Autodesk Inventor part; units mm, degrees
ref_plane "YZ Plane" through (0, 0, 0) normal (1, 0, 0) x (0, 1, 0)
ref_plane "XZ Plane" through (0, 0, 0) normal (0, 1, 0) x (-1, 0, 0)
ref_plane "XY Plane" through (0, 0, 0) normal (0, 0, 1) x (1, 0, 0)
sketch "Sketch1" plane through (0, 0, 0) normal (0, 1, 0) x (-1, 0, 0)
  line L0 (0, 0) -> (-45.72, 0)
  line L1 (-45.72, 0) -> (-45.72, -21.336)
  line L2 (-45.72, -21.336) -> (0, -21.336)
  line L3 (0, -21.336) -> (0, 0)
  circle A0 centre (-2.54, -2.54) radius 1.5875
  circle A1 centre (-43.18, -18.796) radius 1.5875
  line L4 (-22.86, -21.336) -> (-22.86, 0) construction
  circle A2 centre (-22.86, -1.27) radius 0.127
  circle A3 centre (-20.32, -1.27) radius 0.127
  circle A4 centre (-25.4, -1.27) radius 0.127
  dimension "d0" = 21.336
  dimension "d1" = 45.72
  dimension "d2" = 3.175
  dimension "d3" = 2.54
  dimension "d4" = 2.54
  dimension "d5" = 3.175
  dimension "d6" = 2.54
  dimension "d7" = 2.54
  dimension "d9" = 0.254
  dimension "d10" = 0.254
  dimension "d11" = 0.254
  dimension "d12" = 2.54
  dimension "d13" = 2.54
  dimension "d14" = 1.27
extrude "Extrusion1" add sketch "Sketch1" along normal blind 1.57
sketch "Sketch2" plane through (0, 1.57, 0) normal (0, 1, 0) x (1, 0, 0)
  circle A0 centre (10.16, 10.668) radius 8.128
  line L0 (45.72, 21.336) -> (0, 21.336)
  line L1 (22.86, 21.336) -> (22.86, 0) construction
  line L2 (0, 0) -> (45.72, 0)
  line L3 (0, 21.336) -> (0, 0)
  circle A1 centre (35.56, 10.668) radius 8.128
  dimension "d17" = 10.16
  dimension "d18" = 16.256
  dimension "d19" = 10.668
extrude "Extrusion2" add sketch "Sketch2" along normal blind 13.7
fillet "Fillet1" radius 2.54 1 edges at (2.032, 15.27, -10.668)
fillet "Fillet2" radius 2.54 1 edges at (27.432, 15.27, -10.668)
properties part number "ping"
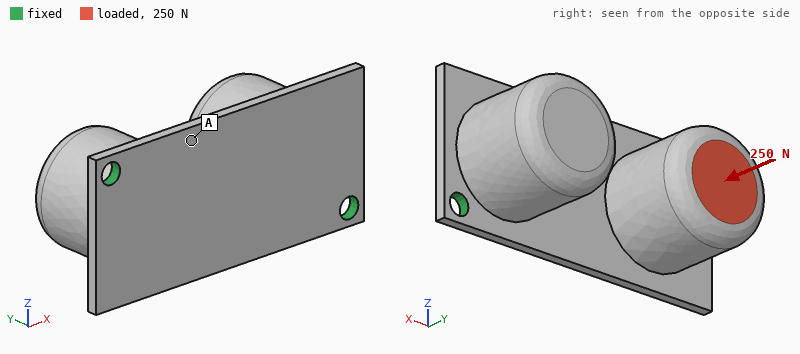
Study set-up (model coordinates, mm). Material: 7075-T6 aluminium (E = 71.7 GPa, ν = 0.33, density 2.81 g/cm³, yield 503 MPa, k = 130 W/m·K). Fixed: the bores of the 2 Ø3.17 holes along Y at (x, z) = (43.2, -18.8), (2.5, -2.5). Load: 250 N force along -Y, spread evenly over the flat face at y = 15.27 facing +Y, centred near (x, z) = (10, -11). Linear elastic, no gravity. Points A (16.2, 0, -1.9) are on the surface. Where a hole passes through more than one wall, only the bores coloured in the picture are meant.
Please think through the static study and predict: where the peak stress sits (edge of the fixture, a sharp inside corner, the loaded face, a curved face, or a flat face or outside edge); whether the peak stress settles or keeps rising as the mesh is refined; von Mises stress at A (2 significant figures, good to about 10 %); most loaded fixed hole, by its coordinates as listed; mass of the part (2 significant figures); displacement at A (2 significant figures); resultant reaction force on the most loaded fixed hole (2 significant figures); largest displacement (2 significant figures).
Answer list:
edge of the fixture
keeps rising
16 MPa
(2.5, -2.5)
20 g
0.035 mm
200 N
0.16 mm
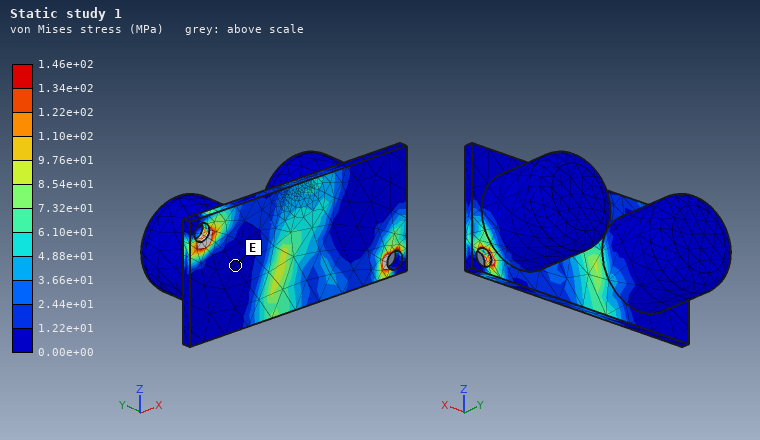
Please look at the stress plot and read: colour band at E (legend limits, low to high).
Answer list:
0.00e+00 to 1.22e+01 MPa
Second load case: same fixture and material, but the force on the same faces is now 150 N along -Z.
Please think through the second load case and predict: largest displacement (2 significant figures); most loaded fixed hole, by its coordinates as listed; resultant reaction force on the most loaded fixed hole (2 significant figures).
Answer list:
0.19 mm
(2.5, -2.5)
130 N
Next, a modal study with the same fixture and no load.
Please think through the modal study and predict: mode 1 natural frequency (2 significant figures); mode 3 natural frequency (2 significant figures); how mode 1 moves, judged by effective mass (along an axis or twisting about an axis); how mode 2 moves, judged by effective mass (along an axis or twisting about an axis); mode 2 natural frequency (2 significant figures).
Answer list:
1800 Hz
3300 Hz
along Y
along Z
2000 Hz
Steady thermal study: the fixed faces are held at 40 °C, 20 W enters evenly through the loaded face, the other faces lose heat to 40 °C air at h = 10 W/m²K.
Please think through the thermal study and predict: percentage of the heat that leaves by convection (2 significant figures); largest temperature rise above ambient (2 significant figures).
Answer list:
3.7 %
45 K
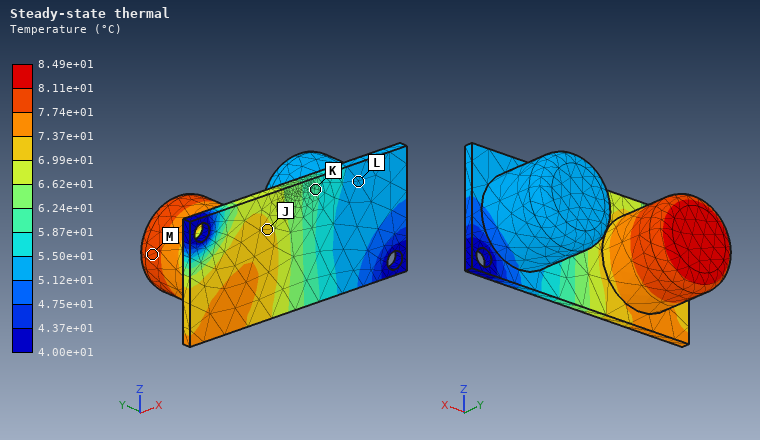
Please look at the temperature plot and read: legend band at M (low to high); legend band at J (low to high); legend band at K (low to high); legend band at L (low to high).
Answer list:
7.74e+01 to 8.11e+01 °C
6.99e+01 to 7.37e+01 °C
5.87e+01 to 6.24e+01 °C
5.12e+01 to 5.50e+01 °C
